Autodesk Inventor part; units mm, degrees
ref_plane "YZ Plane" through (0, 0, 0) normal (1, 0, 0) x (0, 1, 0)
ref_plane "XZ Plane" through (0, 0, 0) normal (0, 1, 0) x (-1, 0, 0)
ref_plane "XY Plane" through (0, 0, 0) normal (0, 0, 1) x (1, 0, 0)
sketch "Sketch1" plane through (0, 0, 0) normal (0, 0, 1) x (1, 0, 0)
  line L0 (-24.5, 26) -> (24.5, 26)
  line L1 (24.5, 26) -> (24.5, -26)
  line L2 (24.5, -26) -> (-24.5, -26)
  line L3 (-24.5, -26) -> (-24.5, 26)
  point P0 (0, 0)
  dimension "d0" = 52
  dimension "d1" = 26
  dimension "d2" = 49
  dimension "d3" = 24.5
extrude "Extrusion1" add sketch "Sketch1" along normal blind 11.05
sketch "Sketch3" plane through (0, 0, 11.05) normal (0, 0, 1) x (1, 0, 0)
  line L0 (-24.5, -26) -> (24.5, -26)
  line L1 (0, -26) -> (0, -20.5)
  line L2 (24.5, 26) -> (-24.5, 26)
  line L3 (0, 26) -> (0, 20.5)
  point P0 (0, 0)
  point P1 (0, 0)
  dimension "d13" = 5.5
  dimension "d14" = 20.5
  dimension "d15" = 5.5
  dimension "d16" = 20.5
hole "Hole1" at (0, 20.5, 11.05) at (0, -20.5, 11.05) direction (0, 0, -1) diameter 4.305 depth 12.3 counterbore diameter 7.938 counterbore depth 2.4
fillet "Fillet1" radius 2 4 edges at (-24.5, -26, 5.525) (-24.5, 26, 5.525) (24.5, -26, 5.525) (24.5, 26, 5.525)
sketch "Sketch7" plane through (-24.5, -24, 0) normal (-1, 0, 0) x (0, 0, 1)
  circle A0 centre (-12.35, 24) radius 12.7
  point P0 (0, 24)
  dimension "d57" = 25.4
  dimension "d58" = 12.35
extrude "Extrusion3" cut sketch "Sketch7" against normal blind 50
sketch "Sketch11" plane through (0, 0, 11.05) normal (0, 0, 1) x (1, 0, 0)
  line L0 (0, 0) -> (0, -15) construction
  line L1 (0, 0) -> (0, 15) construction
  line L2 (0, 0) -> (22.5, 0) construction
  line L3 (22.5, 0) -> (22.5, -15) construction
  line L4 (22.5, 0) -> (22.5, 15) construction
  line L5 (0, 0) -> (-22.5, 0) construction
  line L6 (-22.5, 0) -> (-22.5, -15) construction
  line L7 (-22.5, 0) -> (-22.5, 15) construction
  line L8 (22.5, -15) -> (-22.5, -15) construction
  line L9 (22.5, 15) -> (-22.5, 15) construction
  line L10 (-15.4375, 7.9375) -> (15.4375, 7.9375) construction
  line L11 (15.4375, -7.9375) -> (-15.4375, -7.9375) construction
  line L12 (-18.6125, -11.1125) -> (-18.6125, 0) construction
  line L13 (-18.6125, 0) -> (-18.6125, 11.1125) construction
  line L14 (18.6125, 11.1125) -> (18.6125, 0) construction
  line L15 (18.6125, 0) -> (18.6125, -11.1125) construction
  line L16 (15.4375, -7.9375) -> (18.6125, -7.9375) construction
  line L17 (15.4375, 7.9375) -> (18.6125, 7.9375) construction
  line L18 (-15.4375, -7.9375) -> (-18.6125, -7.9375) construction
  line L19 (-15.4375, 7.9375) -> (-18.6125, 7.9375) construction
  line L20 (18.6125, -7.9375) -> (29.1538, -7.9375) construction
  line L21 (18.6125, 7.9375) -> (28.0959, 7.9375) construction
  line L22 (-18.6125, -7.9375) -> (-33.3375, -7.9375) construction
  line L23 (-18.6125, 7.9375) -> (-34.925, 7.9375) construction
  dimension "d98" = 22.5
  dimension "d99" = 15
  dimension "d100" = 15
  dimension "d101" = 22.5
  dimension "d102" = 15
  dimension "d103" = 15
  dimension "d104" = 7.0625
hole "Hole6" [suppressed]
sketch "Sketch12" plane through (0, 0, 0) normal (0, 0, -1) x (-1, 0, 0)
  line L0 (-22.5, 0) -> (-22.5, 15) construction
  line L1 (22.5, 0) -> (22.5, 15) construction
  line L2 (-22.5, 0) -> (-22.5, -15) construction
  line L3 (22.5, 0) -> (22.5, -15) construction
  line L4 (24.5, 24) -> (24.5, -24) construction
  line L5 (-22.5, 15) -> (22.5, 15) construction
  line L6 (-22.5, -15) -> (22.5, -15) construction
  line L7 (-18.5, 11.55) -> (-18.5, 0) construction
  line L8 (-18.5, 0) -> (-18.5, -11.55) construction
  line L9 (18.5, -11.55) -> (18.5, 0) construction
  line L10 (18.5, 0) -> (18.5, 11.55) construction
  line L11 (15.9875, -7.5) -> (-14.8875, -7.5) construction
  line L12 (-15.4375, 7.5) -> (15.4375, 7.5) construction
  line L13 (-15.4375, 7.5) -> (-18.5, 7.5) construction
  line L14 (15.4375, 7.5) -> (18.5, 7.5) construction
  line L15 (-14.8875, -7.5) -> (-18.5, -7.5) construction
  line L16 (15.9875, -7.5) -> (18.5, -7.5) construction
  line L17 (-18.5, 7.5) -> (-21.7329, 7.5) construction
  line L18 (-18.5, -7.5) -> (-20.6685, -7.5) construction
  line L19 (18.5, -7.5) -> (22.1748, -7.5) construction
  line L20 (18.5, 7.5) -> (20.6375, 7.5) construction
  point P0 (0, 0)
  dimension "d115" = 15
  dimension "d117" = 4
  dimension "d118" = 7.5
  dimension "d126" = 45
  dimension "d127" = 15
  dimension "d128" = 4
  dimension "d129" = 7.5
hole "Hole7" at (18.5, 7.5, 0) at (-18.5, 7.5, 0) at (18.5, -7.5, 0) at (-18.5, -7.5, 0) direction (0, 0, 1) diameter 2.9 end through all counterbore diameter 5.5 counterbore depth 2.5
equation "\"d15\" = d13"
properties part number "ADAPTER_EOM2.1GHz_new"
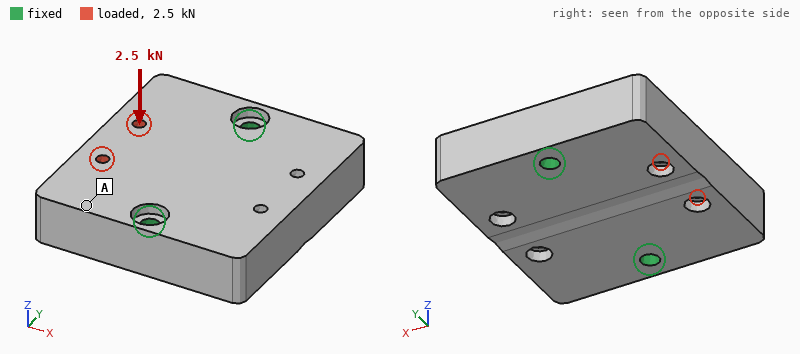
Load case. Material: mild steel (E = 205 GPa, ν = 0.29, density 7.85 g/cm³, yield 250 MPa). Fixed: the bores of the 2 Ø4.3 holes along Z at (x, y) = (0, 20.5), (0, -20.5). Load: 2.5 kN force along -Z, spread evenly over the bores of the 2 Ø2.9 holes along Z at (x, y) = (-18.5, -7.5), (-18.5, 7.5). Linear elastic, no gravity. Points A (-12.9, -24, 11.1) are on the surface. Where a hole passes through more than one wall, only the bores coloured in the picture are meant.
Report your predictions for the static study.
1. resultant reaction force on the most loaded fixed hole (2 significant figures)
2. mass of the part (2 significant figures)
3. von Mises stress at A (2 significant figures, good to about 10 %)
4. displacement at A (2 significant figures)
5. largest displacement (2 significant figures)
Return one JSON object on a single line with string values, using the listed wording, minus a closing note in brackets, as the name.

{"resultant reaction force on the most loaded fixed hole": "1.3 kN", "mass of the part": "210 g", "von Mises stress at A": "19 MPa", "displacement at A": "7.5 µm", "largest displacement": "21 µm"}
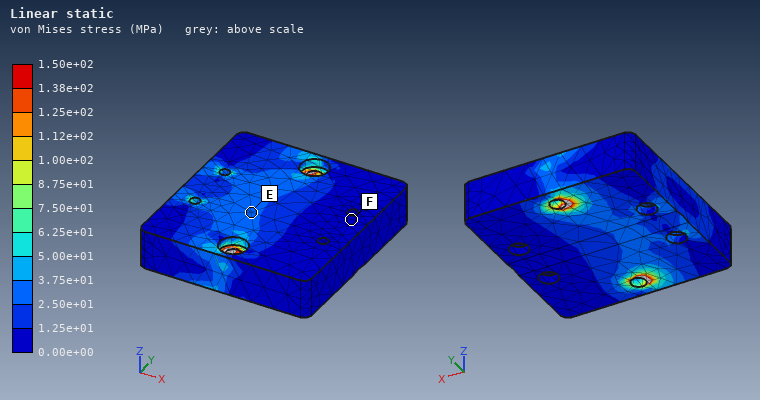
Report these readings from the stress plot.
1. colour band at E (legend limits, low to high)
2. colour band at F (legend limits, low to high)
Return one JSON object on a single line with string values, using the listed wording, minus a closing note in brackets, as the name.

{"colour band at E": "2.50e+01 to 3.75e+01 MPa", "colour band at F": "0.00e+00 to 1.25e+01 MPa"}
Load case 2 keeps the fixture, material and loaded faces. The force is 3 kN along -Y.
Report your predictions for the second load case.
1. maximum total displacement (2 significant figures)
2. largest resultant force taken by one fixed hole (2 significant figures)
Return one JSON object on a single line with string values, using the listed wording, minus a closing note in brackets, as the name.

{"maximum total displacement": "2.5 µm", "largest resultant force taken by one fixed hole": "2.0 kN"}
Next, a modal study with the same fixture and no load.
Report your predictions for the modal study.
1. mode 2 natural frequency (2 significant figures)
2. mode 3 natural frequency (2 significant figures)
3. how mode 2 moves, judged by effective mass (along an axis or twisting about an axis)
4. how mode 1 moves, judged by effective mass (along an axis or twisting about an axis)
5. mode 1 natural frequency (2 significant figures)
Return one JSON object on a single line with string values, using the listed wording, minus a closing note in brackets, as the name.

{"mode 2 natural frequency": "11 kHz", "mode 3 natural frequency": "16 kHz", "how mode 2 moves, judged by effective mass": "along Z", "how mode 1 moves, judged by effective mass": "twisting about Y", "mode 1 natural frequency": "7400 Hz"}
